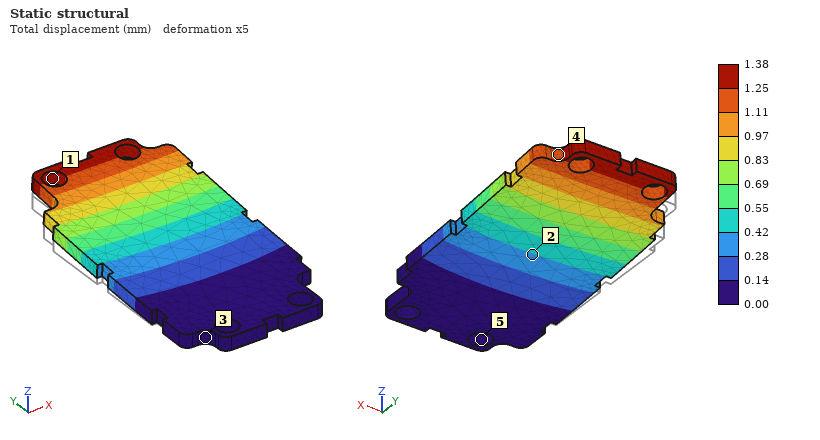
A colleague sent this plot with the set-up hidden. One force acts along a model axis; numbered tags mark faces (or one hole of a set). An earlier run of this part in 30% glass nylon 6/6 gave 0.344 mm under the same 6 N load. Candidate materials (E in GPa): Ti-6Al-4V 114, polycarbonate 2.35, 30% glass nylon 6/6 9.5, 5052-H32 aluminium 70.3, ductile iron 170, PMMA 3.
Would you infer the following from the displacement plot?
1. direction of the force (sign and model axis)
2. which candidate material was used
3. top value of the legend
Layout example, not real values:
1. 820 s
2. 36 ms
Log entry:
1. +Z
2. polycarbonate
3. 1.38 mm
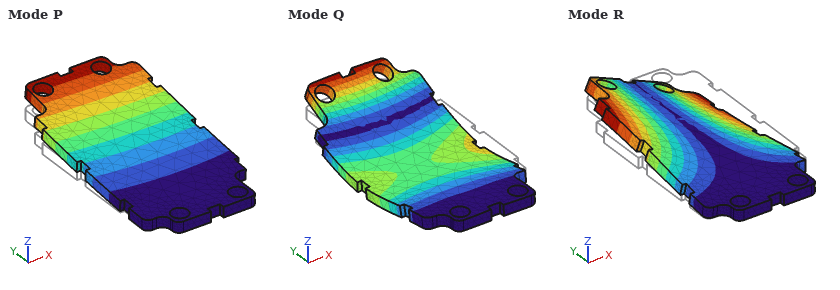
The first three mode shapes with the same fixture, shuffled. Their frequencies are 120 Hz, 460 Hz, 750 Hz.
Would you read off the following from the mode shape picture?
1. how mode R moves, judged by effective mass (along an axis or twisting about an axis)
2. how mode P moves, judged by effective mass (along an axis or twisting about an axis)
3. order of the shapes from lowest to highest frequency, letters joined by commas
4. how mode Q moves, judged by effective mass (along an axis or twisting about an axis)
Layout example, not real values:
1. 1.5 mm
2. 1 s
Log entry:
1. twisting about Y
2. along Z
3. P, R, Q
4. along Z
